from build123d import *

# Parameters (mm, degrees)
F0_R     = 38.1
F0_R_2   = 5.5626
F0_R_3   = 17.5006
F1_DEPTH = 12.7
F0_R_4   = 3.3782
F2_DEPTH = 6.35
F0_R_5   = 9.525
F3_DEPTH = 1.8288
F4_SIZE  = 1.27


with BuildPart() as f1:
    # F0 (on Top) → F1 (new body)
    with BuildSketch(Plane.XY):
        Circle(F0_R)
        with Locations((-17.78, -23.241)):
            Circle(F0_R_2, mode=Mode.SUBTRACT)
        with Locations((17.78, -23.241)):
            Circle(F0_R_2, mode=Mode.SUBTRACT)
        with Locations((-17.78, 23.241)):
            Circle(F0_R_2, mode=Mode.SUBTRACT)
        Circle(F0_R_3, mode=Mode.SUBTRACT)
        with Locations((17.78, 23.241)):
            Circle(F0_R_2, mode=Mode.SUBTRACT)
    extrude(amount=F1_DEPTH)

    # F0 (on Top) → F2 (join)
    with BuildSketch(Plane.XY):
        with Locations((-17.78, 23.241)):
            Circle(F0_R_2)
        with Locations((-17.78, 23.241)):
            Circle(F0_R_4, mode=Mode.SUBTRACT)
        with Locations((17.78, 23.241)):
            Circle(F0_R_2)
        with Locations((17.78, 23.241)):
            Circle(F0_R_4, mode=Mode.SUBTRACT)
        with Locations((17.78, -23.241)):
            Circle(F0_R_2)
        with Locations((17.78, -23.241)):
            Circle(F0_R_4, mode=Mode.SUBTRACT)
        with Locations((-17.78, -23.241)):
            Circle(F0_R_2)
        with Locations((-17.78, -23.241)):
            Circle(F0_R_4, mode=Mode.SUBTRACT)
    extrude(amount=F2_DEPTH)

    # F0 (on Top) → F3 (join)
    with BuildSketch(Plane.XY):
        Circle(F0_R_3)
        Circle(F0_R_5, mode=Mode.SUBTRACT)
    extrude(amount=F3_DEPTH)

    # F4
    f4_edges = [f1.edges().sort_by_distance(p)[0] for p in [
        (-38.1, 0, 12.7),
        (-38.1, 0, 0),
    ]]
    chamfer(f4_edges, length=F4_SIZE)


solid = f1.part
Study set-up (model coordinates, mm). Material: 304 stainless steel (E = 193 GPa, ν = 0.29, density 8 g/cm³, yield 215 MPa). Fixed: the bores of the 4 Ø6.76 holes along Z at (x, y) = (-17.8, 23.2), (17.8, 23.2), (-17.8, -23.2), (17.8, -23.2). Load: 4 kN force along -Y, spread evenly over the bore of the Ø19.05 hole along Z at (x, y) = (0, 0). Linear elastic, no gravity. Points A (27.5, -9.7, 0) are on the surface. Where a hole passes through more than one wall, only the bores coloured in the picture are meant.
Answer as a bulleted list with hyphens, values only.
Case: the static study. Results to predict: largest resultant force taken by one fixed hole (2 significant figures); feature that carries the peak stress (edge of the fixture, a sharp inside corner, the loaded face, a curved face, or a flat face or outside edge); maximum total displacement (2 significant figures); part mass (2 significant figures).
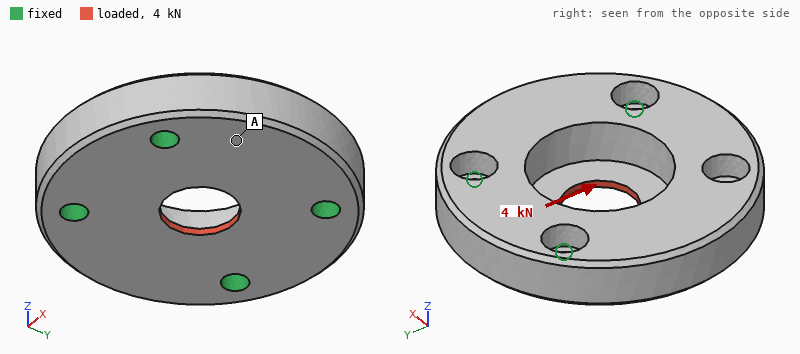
- 1.0 kN
- the loaded face
- 3.3 µm
- 350 g
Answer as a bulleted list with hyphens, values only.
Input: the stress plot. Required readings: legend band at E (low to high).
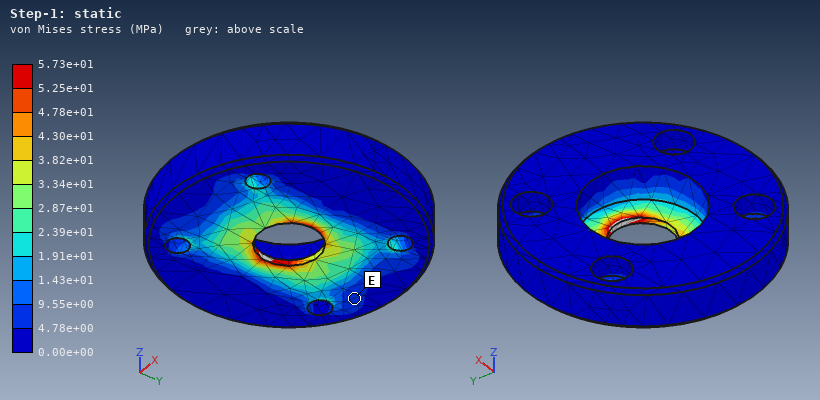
- 4.78e+00 to 9.55e+00 MPa
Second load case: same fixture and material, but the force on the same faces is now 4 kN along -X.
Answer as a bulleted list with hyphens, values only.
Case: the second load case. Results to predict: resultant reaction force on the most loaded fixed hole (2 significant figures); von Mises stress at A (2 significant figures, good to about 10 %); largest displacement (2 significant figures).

- 1.0 kN
- 6.6 MPa
- 3.9 µm
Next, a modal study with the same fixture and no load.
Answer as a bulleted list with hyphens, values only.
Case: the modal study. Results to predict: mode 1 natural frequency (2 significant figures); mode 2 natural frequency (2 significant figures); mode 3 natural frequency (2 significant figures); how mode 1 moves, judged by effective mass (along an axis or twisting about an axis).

- 12 kHz
- 12 kHz
- 20 kHz
- along Z
